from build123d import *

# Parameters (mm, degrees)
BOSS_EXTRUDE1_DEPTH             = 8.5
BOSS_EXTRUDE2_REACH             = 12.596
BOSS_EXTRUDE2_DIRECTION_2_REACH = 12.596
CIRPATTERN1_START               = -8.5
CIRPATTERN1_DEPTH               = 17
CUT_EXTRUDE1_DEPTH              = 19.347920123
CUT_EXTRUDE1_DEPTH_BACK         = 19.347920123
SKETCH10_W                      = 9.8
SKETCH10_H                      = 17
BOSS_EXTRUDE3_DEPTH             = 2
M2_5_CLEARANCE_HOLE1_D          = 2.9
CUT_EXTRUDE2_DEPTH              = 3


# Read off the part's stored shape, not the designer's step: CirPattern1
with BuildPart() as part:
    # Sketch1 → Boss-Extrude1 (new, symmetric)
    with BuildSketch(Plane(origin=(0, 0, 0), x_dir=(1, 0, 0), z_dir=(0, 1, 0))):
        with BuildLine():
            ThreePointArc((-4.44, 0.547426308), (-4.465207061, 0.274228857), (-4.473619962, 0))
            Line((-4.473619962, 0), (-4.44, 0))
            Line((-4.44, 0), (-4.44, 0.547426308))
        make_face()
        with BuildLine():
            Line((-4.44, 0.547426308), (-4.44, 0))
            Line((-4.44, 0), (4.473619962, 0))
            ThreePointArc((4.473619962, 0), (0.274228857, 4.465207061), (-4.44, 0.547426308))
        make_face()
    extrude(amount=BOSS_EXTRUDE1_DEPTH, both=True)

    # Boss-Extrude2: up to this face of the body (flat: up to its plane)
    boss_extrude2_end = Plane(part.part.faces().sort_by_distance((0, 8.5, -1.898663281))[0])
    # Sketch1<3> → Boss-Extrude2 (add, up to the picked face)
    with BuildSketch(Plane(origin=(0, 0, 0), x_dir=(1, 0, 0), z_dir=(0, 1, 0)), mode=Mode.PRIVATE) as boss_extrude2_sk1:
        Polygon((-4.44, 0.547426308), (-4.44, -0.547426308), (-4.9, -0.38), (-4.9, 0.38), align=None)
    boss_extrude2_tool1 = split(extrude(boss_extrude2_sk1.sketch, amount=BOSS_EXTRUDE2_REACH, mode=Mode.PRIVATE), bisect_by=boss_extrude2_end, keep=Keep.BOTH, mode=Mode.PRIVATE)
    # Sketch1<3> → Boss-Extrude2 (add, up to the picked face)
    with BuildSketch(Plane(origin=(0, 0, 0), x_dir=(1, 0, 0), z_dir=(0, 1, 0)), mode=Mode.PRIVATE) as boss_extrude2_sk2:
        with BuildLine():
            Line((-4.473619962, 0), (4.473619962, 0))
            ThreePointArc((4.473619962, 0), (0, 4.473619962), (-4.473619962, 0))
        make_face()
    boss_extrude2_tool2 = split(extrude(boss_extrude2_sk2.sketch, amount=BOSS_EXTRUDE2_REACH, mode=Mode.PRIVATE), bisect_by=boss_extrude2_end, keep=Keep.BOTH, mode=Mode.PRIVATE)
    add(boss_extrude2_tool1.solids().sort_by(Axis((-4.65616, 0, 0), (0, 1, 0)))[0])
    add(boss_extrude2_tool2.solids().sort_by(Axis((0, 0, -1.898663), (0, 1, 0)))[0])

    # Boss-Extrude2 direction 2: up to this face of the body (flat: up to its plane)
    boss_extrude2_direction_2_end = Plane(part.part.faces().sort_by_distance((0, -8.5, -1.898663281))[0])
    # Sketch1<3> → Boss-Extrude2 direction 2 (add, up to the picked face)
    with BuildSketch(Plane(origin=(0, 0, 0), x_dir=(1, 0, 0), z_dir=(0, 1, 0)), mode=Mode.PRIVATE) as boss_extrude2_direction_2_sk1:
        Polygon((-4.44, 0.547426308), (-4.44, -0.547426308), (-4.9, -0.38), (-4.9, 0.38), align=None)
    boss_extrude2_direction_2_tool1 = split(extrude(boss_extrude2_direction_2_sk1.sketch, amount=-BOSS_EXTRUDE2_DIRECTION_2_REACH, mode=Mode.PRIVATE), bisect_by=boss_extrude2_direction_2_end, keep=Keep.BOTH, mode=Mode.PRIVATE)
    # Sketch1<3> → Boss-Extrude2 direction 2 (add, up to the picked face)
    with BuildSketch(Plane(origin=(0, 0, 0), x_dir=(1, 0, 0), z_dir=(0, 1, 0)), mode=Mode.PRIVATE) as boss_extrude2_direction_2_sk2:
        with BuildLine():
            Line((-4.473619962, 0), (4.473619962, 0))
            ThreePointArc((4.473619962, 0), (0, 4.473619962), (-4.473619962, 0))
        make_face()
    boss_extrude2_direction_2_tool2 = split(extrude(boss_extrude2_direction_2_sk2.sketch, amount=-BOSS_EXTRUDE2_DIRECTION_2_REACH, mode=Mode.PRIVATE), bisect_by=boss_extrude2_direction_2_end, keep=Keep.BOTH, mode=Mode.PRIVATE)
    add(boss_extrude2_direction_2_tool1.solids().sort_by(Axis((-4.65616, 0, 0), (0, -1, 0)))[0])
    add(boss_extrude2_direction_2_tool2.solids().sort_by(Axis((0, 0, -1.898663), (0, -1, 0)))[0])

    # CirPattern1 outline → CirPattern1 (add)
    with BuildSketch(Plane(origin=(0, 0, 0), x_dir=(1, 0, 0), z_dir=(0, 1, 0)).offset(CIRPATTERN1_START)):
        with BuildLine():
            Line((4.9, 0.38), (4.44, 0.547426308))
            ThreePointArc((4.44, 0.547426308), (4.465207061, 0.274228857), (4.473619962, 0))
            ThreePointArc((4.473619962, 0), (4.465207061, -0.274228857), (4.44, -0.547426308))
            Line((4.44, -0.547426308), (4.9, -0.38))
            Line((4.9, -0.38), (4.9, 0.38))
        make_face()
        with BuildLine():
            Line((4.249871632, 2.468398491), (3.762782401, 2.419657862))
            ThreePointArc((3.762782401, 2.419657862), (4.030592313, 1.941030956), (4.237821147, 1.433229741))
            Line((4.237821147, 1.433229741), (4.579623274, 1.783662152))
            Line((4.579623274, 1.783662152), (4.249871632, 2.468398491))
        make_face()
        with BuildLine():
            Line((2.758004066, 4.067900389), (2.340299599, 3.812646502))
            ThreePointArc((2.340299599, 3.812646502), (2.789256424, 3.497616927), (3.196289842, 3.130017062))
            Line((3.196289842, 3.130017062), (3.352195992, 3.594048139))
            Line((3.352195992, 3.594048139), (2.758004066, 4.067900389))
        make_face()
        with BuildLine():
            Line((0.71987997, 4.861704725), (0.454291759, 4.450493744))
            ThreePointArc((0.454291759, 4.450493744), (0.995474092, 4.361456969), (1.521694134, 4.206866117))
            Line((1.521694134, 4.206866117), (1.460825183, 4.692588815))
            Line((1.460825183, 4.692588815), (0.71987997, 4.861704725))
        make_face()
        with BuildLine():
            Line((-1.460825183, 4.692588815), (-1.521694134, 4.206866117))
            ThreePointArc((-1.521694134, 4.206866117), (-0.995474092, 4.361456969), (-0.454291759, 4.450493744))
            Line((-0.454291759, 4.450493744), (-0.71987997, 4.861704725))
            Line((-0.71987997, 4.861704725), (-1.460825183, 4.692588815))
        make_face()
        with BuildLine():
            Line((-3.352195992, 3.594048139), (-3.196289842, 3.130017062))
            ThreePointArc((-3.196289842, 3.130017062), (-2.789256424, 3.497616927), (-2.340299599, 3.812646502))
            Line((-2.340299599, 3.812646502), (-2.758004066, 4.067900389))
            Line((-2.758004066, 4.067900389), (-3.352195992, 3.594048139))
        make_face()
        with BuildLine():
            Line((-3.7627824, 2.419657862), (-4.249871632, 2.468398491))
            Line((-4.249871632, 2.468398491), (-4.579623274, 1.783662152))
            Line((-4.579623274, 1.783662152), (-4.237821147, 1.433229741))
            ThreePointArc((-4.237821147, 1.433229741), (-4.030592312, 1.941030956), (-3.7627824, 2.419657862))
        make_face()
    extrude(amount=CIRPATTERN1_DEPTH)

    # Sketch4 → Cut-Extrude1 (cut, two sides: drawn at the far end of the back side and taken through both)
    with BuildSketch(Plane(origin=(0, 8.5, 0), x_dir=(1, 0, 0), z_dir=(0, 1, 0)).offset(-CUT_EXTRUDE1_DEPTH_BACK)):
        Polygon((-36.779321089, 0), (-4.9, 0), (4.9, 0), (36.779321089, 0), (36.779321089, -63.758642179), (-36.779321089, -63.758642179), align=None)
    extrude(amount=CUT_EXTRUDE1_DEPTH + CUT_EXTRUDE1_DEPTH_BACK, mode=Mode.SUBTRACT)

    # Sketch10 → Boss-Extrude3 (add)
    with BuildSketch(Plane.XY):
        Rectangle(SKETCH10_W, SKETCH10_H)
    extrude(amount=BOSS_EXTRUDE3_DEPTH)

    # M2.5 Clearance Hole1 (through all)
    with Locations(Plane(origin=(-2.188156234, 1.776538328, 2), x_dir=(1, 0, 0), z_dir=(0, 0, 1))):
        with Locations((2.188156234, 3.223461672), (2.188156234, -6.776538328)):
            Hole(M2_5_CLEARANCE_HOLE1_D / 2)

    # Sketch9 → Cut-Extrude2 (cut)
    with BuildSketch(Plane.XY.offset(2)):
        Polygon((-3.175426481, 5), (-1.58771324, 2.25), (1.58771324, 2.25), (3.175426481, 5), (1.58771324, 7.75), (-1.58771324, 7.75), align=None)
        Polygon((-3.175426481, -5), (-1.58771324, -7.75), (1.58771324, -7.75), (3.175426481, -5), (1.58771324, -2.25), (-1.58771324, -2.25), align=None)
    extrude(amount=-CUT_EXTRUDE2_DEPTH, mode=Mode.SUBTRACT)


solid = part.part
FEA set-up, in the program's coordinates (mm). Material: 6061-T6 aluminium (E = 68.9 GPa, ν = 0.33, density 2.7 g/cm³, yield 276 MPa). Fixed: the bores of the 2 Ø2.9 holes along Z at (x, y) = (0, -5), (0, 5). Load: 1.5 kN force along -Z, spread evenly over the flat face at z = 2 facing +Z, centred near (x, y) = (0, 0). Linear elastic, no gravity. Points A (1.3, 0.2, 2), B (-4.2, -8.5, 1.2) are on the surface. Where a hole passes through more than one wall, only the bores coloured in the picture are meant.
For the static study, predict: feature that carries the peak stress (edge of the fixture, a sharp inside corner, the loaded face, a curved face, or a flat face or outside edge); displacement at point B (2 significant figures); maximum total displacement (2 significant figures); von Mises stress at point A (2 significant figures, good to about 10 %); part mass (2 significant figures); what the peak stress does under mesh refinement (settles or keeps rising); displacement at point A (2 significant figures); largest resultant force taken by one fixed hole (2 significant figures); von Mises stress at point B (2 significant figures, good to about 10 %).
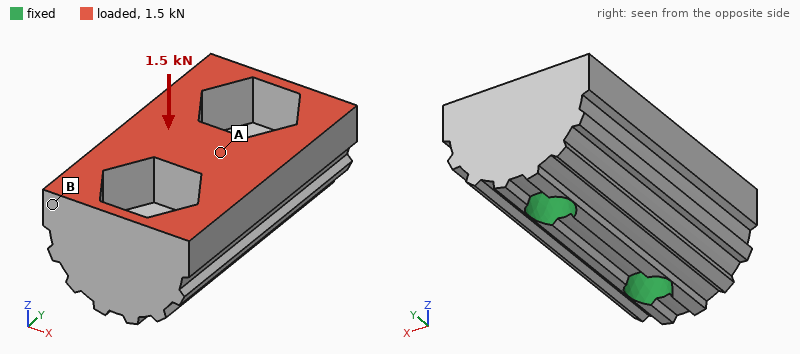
edge of the fixture
2.9 µm
3.8 µm
23 MPa
1.9 g
keeps rising
2.9 µm
760 N
13 MPa
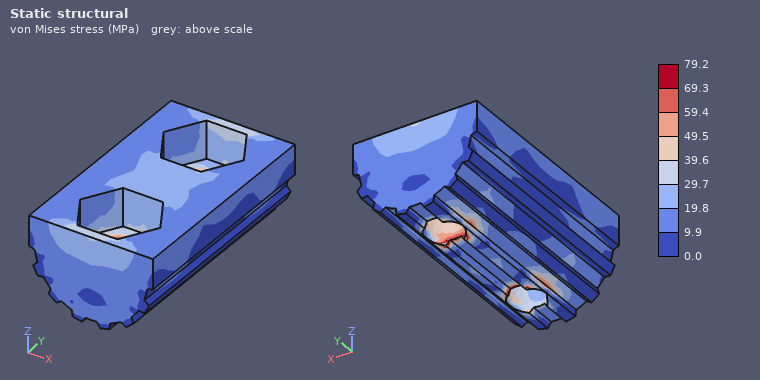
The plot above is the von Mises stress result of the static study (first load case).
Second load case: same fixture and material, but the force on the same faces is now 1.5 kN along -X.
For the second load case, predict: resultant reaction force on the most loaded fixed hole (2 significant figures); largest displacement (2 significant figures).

750 N
21 µm
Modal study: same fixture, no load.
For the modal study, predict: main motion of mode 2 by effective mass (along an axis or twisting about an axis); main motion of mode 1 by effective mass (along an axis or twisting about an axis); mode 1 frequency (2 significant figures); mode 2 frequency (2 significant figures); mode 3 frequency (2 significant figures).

twisting about Z
along X
57 kHz
80 kHz
90 kHz
